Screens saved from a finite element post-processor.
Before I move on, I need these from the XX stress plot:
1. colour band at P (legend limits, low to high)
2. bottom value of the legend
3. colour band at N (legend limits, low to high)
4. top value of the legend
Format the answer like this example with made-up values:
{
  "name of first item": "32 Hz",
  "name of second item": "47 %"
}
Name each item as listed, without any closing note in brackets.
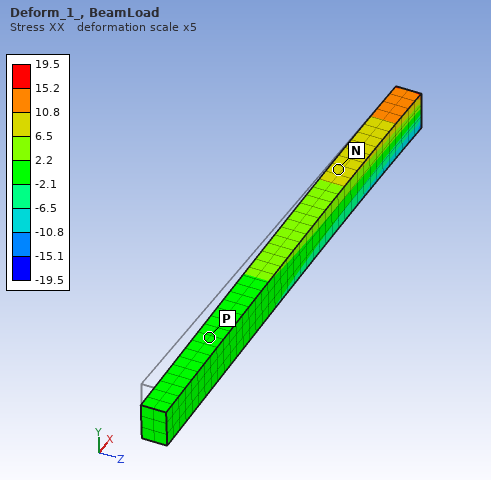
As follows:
{
  "colour band at P": "-2.1 to 2.2",
  "bottom value of the legend": "-19.5",
  "colour band at N": "6.5 to 10.8",
  "top value of the legend": "19.5"
}
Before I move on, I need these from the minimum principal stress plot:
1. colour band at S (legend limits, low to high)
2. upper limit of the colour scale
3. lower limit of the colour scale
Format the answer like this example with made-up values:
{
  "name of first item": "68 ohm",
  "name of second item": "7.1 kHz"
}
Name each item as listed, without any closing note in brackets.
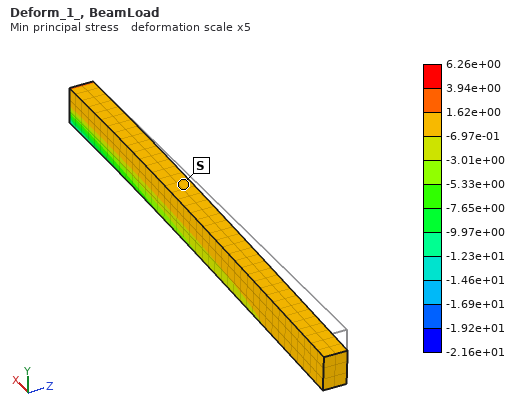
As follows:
{
  "colour band at S": "-6.97e-01 to 1.62e+00",
  "upper limit of the colour scale": "6.26e+00",
  "lower limit of the colour scale": "-2.16e+01"
}
